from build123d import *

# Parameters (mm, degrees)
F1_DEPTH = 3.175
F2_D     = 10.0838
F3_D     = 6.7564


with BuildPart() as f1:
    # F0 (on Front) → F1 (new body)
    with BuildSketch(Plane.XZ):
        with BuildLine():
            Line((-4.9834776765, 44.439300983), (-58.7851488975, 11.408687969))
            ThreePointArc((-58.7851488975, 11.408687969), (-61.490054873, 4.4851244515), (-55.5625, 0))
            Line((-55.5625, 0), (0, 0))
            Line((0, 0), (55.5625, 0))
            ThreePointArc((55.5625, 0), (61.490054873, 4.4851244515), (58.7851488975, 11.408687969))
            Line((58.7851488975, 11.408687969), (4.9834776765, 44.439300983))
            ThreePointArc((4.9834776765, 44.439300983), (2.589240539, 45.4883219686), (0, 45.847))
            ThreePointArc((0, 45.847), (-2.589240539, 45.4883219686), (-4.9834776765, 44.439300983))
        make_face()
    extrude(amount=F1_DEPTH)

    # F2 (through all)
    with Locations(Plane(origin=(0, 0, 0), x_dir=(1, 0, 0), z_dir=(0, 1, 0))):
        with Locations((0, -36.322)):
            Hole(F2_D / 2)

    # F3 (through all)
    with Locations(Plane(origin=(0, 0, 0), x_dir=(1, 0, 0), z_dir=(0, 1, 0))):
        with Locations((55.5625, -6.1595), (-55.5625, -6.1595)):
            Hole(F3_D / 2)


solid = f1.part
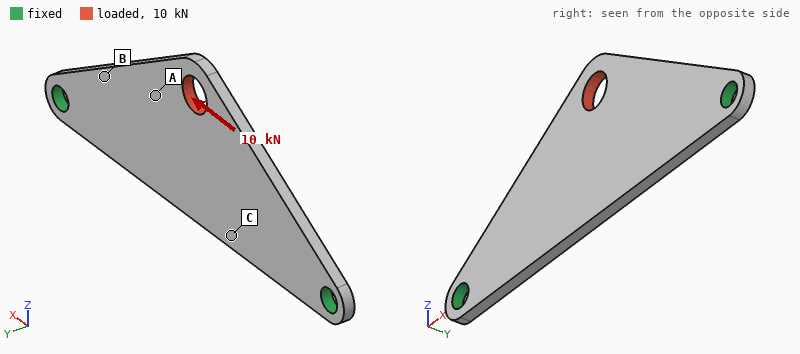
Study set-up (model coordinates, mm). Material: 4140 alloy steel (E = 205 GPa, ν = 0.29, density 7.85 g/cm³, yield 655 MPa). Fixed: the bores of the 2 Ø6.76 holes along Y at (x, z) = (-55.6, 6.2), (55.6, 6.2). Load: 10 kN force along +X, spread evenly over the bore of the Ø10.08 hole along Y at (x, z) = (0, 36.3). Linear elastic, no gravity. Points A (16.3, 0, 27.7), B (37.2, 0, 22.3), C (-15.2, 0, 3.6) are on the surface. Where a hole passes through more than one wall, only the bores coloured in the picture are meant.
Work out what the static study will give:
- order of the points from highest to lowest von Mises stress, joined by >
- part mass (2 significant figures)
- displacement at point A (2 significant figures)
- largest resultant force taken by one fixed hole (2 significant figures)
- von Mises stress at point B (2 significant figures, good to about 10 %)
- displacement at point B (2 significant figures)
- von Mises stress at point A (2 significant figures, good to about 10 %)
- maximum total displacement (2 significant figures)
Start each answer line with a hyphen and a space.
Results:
- B > A > C
- 83 g
- 23 µm
- 5.8 kN
- 130 MPa
- 14 µm
- 86 MPa
- 49 µm
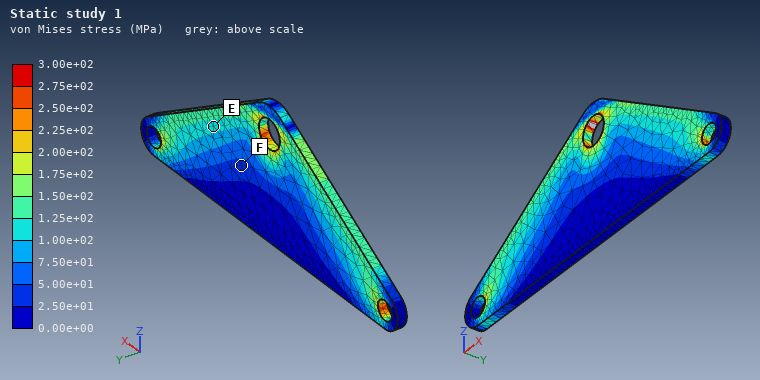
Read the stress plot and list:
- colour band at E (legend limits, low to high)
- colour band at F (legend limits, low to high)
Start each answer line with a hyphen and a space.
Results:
- 1.00e+02 to 1.25e+02 MPa
- 2.50e+01 to 5.00e+01 MPa
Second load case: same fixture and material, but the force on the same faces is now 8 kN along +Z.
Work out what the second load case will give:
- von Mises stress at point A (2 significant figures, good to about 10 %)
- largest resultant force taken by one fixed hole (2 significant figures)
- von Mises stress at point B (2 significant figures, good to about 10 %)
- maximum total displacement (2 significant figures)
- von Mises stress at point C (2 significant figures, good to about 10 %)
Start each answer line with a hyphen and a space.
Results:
- 110 MPa
- 5.8 kN
- 150 MPa
- 75 µm
- 67 MPa
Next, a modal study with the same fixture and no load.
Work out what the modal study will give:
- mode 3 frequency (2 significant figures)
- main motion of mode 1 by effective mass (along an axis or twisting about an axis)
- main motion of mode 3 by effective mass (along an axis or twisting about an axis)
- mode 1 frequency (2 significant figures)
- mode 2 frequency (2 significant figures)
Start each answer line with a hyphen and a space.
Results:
- 3200 Hz
- along Y
- twisting about Z
- 980 Hz
- 2100 Hz
